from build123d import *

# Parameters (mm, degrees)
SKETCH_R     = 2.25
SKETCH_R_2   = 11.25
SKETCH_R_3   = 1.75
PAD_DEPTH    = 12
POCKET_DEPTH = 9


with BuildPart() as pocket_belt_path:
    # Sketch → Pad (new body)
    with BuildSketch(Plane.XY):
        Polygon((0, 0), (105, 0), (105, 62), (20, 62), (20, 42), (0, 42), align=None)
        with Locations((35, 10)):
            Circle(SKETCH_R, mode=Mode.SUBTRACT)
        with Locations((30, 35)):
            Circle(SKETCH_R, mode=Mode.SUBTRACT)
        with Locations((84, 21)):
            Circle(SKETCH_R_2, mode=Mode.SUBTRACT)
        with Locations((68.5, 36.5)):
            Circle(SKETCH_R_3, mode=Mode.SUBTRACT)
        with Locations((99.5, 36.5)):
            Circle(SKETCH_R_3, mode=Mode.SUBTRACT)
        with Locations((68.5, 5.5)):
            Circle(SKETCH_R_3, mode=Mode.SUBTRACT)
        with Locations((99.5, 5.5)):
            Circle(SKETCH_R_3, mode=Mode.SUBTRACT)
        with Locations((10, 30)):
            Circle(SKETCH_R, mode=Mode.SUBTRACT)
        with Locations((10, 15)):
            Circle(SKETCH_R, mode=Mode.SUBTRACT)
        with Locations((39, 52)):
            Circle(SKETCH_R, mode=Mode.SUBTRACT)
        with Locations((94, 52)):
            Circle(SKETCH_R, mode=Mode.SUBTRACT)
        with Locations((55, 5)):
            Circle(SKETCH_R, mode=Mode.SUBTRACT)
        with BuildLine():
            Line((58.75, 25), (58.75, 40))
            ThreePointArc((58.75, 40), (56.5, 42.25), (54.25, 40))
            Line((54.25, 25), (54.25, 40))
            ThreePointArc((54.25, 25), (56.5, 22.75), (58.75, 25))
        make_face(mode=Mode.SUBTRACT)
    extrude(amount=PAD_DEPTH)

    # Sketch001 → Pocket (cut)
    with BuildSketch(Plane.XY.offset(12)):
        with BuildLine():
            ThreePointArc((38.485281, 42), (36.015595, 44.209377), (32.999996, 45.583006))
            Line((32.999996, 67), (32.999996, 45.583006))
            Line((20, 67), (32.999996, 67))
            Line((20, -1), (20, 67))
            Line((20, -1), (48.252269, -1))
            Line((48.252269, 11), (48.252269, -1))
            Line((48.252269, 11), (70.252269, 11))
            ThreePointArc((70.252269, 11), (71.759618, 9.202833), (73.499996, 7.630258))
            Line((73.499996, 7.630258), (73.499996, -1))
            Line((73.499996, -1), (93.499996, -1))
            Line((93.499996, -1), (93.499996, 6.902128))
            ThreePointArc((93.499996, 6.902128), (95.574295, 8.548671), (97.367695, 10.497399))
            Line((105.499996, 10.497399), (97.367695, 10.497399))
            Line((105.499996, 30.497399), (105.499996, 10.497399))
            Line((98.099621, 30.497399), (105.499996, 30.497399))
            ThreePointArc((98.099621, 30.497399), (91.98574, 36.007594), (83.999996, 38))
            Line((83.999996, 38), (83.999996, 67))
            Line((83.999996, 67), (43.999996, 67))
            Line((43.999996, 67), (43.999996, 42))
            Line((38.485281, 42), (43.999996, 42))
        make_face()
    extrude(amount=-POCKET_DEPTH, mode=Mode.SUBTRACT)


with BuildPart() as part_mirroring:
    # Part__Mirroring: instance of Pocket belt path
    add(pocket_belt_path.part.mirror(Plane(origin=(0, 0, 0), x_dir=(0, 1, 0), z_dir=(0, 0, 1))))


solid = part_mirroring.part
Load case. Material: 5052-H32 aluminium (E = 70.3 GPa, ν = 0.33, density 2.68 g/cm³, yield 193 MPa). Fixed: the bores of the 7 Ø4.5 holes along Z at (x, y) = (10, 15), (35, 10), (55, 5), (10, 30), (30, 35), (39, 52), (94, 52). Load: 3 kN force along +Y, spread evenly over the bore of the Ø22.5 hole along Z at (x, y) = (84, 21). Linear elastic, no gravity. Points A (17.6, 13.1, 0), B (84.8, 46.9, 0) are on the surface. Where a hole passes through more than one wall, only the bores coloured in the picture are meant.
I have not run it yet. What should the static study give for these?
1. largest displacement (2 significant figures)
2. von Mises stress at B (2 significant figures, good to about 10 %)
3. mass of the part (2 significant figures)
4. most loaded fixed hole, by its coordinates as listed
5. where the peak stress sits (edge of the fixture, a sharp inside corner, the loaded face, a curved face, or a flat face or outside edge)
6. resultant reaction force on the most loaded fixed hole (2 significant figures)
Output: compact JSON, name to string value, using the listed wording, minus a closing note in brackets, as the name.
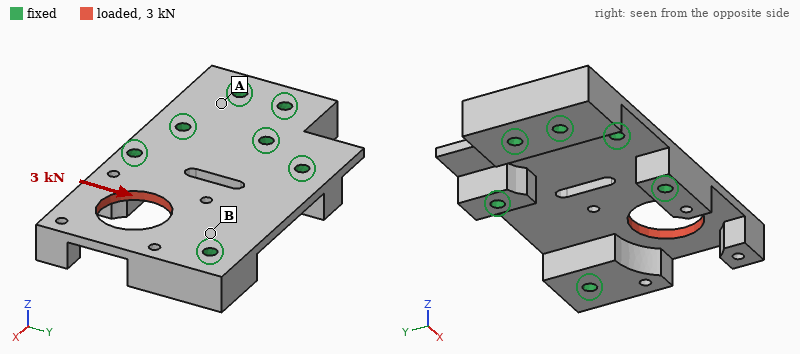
{"largest displacement": "23 µm", "von Mises stress at B": "12 MPa", "mass of the part": "90 g", "most loaded fixed hole, by its coordinates as listed": "(94, 52)", "where the peak stress sits": "the loaded face", "resultant reaction force on the most loaded fixed hole": "1.9 kN"}
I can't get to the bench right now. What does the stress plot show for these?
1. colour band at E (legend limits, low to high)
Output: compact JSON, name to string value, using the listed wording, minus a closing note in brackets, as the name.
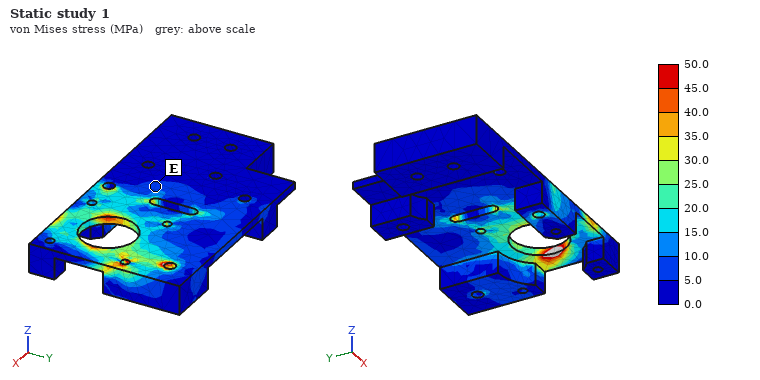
{"colour band at E": "5.0 to 10.0 MPa"}
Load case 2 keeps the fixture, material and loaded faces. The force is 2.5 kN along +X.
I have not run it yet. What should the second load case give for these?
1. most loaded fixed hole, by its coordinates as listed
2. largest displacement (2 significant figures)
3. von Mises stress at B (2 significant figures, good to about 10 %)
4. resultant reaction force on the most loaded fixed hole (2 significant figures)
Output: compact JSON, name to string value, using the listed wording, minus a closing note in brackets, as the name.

{"most loaded fixed hole, by its coordinates as listed": "(55, 5)", "largest displacement": "19 µm", "von Mises stress at B": "7.4 MPa", "resultant reaction force on the most loaded fixed hole": "1.1 kN"}
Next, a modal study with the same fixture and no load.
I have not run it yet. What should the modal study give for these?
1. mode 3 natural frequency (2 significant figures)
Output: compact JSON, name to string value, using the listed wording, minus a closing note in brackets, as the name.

{"mode 3 natural frequency": "8000 Hz"}
